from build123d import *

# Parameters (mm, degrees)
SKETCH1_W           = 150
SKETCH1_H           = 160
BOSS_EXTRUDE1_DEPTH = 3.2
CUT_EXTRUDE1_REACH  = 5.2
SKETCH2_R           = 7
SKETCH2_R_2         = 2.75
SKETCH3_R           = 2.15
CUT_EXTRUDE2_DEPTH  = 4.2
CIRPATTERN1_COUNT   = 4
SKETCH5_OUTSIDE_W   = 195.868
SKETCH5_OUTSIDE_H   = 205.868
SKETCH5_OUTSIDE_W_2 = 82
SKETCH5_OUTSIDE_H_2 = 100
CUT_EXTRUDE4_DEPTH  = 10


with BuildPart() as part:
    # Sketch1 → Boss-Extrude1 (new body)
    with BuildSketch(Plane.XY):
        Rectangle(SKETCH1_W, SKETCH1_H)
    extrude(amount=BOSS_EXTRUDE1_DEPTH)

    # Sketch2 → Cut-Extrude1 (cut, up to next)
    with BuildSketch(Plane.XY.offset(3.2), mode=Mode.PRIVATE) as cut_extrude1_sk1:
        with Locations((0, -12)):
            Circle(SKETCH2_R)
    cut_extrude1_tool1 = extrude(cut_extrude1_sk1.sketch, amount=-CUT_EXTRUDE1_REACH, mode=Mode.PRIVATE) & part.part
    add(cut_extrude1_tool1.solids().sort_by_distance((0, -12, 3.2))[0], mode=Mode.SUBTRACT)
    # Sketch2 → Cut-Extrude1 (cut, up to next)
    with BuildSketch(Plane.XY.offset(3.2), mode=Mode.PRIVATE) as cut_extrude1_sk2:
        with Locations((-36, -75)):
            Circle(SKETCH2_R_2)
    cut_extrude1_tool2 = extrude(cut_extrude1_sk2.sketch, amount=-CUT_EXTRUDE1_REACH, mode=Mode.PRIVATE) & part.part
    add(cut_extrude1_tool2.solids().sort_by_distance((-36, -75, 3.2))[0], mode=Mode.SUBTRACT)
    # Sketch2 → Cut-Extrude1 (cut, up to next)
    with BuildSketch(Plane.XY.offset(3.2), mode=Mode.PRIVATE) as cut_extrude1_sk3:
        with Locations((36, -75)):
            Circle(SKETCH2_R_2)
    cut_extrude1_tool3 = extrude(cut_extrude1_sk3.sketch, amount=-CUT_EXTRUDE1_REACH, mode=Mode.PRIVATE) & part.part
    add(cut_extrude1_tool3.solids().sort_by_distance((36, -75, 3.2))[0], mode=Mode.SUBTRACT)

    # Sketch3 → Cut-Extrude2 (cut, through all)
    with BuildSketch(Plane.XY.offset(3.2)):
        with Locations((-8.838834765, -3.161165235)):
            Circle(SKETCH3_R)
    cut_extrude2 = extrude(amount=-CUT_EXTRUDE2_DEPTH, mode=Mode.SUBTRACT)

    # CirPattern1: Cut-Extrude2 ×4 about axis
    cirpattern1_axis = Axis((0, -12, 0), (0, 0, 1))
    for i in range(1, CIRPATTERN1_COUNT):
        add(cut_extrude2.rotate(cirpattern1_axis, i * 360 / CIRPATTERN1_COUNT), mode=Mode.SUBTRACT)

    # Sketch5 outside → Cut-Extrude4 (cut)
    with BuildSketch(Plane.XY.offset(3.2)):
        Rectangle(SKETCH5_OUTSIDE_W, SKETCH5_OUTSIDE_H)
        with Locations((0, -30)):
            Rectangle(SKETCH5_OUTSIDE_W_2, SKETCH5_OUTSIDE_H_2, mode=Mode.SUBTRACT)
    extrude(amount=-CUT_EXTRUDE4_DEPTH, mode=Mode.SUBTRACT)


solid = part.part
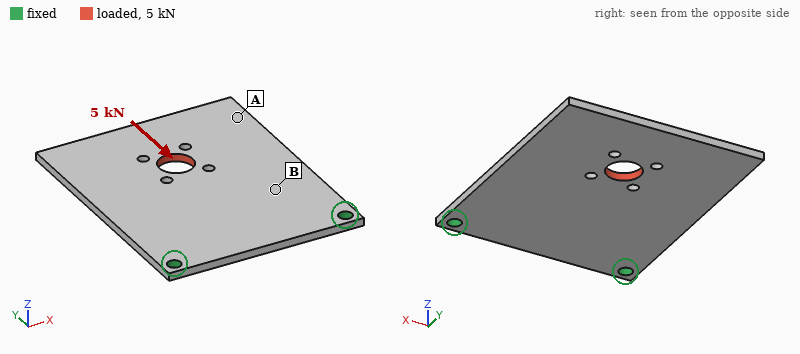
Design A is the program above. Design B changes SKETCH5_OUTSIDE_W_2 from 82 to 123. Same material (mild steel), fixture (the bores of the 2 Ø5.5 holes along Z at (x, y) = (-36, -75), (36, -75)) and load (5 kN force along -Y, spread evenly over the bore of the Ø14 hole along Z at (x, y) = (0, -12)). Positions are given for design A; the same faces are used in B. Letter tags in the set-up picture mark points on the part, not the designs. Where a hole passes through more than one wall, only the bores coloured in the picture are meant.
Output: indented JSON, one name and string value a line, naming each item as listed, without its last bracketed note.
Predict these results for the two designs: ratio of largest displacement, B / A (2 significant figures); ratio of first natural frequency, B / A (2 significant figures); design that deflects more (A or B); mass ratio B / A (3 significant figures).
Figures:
{
  "ratio of largest displacement, B / A": "0.90",
  "ratio of first natural frequency, B / A": "1.0",
  "design that deflects more": "A",
  "mass ratio B / A": "1.52"
}
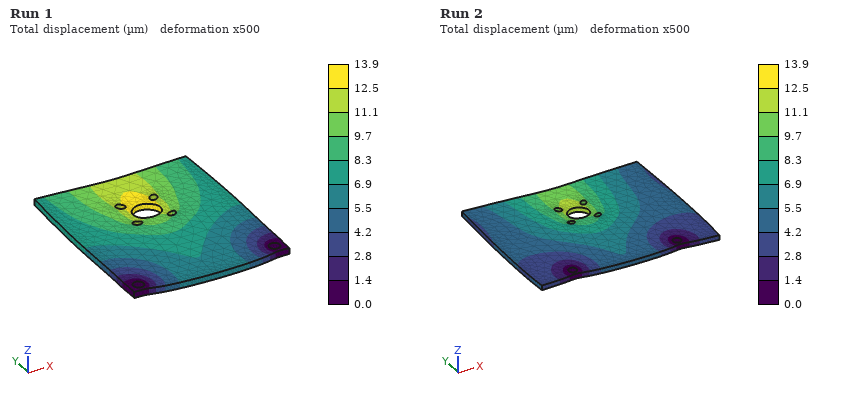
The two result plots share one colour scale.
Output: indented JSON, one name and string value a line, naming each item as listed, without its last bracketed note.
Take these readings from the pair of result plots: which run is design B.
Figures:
{
  "which run is design B": "Run 2"
}
